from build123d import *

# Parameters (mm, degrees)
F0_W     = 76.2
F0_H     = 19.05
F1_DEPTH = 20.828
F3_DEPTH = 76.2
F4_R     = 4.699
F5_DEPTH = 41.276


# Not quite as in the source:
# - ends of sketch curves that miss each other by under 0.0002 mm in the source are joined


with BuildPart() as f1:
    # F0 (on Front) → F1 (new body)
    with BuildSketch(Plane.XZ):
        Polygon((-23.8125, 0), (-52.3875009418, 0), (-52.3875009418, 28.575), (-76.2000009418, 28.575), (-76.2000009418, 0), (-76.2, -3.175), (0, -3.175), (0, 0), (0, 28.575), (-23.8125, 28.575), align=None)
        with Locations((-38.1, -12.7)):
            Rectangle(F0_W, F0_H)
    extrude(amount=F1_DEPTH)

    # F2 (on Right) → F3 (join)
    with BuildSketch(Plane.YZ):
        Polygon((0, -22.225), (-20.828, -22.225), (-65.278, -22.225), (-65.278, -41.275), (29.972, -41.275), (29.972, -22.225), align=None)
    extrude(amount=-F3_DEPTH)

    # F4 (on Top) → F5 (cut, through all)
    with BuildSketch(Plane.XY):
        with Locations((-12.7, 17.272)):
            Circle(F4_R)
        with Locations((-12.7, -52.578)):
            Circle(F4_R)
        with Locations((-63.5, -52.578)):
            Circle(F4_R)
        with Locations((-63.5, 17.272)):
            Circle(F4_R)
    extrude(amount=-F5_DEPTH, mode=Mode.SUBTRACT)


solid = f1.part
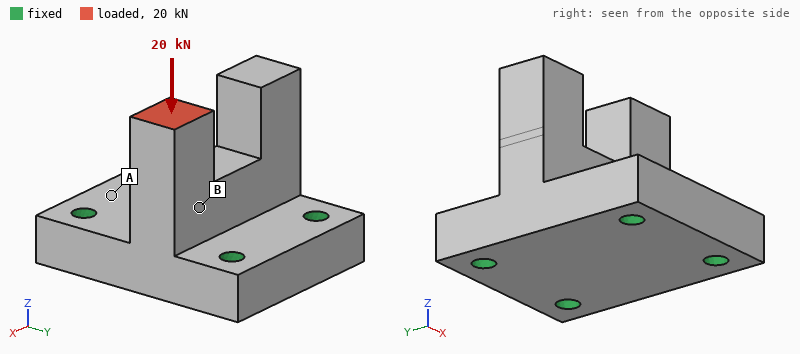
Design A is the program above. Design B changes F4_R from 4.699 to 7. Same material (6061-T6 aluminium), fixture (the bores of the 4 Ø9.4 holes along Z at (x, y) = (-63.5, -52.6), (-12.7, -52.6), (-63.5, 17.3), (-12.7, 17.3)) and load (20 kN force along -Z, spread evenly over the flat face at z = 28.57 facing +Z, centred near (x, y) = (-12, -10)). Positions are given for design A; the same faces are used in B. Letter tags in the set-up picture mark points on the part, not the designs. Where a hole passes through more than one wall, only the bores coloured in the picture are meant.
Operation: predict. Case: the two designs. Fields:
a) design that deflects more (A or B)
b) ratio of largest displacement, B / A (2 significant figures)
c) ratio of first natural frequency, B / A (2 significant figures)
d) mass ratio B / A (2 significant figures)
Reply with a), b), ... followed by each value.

a) A
b) 0.90
c) 1.0
d) 0.97
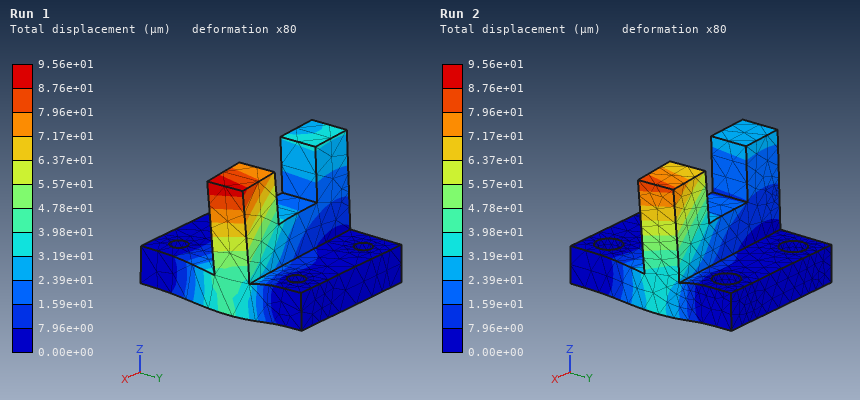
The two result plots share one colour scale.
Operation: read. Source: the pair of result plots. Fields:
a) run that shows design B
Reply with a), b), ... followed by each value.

a) Run 2
